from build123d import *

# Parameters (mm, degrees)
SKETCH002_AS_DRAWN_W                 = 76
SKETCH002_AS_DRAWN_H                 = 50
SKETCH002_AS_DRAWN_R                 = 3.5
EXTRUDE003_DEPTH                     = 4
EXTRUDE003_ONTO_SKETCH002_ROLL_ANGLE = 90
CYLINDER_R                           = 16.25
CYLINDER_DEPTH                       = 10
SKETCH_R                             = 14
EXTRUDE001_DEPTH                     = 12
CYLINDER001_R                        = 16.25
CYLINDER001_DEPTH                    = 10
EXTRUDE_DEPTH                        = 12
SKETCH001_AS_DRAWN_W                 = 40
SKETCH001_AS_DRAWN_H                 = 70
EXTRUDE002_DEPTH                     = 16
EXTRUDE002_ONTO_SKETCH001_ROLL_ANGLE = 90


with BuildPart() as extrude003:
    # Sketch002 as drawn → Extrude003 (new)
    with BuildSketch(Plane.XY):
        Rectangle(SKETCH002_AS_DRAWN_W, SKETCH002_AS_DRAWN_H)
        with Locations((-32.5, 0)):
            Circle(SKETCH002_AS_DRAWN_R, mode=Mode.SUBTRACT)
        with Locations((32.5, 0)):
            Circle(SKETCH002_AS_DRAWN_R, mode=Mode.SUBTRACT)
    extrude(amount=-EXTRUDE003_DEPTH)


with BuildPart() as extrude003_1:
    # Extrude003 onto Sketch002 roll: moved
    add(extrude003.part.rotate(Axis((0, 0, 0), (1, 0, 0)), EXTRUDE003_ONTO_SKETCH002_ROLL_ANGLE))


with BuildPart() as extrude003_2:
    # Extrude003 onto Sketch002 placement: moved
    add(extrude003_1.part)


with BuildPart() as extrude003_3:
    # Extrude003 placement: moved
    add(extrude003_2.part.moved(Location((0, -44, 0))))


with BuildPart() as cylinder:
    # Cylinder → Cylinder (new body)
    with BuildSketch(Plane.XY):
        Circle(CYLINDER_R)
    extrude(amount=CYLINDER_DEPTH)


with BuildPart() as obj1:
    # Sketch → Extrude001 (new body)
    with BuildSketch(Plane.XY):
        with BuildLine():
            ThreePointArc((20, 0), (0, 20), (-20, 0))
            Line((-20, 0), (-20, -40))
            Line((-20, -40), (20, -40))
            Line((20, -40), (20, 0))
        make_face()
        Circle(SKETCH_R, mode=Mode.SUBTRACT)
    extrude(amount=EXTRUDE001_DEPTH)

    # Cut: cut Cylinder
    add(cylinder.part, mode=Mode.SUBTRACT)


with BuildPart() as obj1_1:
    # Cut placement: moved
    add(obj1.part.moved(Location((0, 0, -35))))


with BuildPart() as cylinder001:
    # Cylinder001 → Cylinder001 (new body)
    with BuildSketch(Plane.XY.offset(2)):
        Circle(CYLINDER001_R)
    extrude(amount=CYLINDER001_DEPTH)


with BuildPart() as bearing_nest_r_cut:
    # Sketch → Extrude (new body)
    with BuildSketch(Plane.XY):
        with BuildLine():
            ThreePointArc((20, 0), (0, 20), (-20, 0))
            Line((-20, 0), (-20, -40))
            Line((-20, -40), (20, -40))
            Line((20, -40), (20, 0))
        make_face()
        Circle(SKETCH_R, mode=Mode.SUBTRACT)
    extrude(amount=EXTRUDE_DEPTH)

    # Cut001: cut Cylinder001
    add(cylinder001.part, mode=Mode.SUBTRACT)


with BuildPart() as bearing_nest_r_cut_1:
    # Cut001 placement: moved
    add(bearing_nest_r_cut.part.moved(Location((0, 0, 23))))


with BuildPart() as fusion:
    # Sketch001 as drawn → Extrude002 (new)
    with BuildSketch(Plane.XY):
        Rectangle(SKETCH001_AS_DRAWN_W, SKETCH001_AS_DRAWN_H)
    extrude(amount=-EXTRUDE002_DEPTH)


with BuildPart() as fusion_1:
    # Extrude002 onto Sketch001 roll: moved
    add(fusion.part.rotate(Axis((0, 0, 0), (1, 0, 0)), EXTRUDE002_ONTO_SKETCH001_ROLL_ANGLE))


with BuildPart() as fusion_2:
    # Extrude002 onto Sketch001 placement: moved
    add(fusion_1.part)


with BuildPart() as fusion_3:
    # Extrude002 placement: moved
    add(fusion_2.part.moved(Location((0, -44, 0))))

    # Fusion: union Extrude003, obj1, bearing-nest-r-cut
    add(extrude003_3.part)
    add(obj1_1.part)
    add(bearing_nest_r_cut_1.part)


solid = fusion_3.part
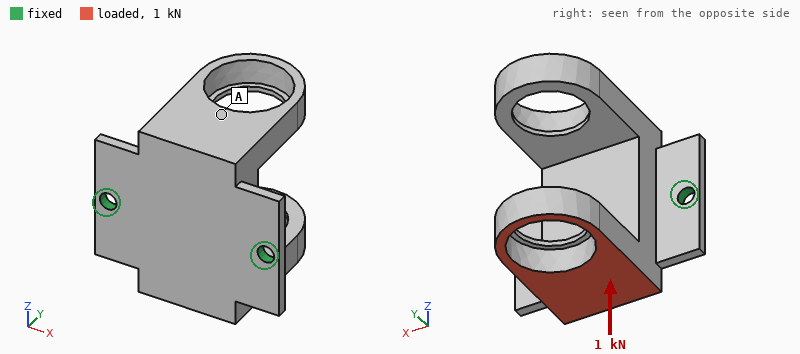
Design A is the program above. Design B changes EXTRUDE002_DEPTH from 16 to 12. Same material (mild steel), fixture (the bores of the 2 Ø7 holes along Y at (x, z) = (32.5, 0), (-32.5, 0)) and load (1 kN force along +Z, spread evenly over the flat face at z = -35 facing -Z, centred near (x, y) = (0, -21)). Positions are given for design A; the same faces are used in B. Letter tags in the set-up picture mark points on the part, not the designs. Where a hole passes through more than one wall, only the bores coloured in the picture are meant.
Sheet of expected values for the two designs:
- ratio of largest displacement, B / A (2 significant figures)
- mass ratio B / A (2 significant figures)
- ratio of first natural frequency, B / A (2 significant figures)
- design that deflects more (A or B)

1.1
0.90
0.99
B
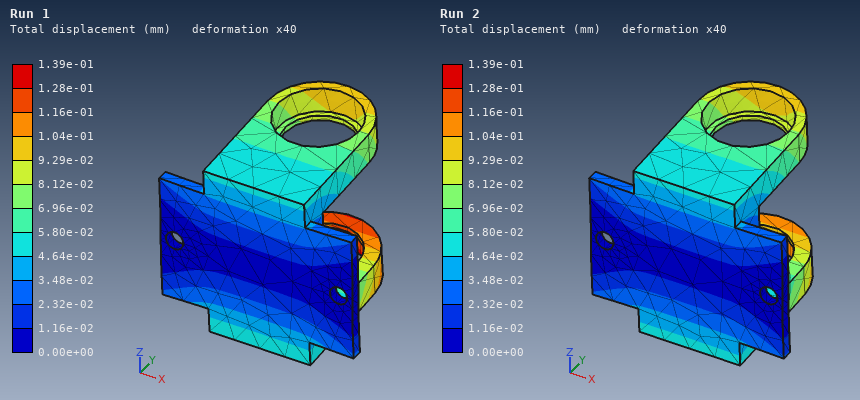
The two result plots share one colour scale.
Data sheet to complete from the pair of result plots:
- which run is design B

Run 1
